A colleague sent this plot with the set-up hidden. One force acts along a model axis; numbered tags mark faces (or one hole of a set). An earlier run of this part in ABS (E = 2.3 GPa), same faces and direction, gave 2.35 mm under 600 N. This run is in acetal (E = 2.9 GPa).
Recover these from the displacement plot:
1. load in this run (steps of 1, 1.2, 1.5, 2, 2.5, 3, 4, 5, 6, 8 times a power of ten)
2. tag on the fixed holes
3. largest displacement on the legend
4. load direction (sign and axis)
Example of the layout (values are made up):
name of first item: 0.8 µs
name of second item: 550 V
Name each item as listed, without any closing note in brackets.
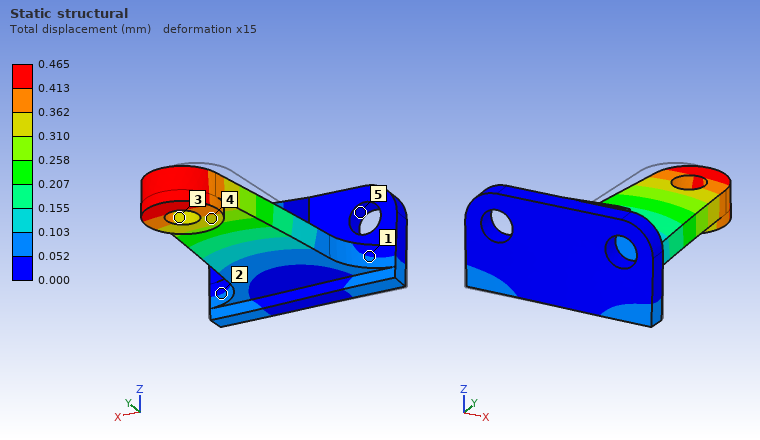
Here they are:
load in this run: 150 N
tag on the fixed holes: 5
largest displacement on the legend: 0.465 mm
load direction: +X
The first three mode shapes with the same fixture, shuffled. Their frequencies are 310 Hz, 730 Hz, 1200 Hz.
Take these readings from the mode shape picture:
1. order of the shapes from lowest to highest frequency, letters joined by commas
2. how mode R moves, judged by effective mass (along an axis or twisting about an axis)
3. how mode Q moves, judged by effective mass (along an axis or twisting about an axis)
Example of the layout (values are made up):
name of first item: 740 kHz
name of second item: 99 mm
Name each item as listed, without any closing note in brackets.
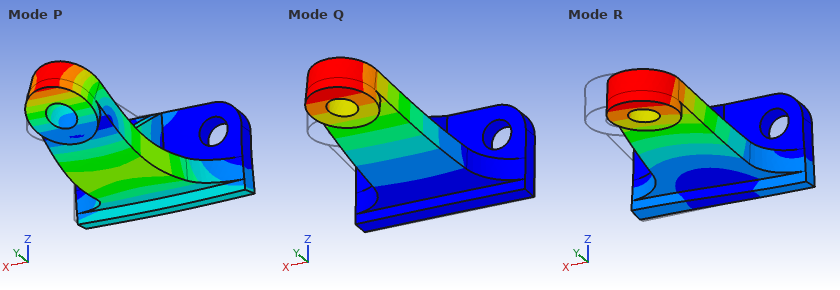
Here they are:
order of the shapes from lowest to highest frequency, letters joined by commas: Q, R, P
how mode R moves, judged by effective mass: along X
how mode Q moves, judged by effective mass: along Z
